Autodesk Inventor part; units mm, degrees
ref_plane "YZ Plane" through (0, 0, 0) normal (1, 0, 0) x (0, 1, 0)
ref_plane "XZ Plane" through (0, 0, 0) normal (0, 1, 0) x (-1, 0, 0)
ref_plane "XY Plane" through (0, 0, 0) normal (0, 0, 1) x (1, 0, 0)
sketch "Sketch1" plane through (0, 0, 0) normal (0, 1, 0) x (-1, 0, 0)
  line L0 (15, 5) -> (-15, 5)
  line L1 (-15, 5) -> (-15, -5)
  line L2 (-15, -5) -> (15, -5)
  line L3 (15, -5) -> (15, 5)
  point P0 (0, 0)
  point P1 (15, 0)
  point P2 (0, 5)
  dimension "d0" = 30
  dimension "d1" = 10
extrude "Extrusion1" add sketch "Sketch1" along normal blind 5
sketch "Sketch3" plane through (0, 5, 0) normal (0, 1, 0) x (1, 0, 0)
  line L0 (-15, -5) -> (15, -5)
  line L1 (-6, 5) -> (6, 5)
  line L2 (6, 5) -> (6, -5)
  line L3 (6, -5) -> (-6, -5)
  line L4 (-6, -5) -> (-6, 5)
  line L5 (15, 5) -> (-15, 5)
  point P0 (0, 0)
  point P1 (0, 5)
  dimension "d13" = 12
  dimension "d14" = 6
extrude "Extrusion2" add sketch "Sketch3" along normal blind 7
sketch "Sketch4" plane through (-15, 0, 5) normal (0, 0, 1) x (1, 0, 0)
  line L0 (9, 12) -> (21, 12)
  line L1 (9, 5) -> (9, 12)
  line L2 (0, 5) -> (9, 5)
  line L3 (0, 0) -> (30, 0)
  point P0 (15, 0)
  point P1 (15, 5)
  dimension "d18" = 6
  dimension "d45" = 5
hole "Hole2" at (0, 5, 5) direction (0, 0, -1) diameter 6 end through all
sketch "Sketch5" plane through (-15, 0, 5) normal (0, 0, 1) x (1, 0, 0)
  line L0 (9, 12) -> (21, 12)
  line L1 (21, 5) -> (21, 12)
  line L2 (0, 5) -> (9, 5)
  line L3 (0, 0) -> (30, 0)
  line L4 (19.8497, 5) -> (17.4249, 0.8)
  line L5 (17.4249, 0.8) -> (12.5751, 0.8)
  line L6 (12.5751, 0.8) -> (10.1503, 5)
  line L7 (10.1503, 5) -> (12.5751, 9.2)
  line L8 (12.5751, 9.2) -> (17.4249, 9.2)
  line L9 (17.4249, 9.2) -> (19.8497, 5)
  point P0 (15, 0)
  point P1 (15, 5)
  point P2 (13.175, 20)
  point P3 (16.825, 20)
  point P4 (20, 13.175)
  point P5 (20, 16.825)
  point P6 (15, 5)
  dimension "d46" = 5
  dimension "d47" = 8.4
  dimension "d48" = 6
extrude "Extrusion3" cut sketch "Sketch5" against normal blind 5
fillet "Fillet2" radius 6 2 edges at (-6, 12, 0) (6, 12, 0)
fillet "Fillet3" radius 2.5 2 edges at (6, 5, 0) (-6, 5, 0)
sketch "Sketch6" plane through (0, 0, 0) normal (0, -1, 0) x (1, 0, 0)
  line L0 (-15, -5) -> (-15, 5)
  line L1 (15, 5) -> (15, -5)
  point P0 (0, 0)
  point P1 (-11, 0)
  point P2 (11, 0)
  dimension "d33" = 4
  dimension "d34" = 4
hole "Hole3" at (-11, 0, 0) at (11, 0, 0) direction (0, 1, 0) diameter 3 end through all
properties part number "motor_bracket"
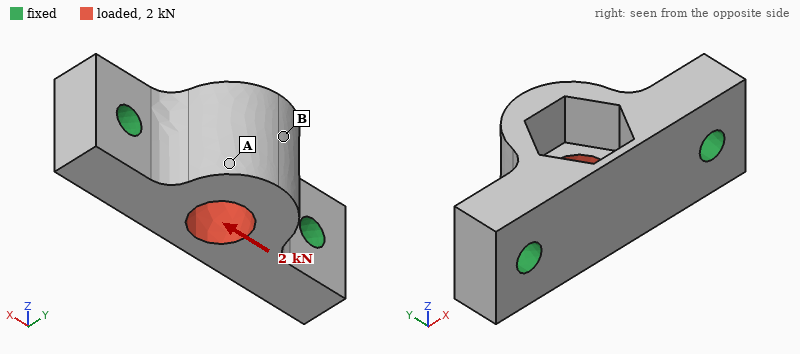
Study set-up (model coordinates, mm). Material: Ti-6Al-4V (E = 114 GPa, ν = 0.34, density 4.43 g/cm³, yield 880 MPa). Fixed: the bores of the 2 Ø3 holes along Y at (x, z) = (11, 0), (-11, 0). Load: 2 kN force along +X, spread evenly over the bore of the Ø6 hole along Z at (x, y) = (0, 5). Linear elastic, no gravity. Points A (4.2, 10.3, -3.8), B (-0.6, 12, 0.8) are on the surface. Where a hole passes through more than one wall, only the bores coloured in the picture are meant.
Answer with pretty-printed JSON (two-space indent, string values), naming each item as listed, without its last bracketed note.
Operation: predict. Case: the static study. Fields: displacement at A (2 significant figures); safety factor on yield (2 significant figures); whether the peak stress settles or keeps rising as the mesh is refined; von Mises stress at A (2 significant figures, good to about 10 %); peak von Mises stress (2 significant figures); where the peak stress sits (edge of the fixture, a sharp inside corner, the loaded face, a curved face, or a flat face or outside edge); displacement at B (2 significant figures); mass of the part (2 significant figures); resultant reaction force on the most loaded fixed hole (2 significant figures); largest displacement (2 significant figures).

{
  "displacement at A": "4.6 µm",
  "safety factor on yield": "11",
  "whether the peak stress settles or keeps rising as the mesh is refined": "settles",
  "von Mises stress at A": "21 MPa",
  "peak von Mises stress": "82 MPa",
  "where the peak stress sits": "a curved face",
  "displacement at B": "3.0 µm",
  "mass of the part": "7.5 g",
  "resultant reaction force on the most loaded fixed hole": "1.0 kN",
  "largest displacement": "5.3 µm"
}
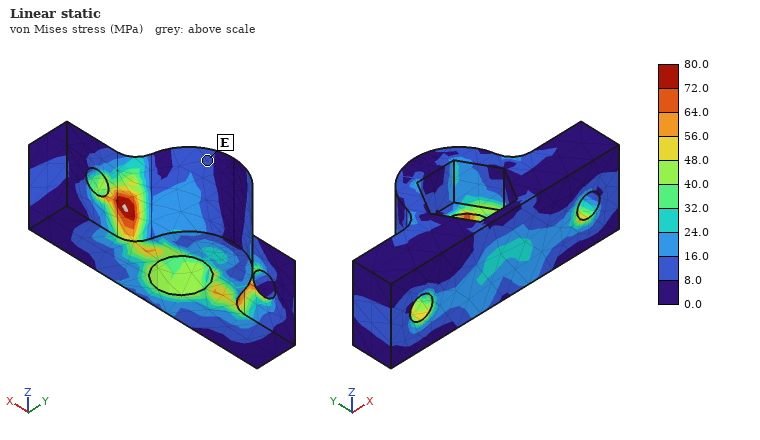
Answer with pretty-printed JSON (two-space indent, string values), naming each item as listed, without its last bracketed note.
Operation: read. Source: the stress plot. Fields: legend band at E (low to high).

{
  "legend band at E": "8.0 to 16.0 MPa"
}
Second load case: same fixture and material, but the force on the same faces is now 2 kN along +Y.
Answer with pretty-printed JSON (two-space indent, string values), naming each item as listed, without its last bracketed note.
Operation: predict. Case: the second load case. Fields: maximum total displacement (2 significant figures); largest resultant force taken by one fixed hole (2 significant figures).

{
  "maximum total displacement": "16 µm",
  "largest resultant force taken by one fixed hole": "1.0 kN"
}
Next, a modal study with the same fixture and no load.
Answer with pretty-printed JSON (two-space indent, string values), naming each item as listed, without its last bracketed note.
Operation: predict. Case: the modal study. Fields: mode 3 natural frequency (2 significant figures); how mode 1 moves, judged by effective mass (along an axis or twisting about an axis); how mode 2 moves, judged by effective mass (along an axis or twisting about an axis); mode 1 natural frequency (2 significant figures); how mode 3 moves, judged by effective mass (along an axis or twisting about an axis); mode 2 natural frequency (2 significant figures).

{
  "mode 3 natural frequency": "51 kHz",
  "how mode 1 moves, judged by effective mass": "along Z",
  "how mode 2 moves, judged by effective mass": "along Y",
  "mode 1 natural frequency": "27 kHz",
  "how mode 3 moves, judged by effective mass": "along Z",
  "mode 2 natural frequency": "45 kHz"
}
